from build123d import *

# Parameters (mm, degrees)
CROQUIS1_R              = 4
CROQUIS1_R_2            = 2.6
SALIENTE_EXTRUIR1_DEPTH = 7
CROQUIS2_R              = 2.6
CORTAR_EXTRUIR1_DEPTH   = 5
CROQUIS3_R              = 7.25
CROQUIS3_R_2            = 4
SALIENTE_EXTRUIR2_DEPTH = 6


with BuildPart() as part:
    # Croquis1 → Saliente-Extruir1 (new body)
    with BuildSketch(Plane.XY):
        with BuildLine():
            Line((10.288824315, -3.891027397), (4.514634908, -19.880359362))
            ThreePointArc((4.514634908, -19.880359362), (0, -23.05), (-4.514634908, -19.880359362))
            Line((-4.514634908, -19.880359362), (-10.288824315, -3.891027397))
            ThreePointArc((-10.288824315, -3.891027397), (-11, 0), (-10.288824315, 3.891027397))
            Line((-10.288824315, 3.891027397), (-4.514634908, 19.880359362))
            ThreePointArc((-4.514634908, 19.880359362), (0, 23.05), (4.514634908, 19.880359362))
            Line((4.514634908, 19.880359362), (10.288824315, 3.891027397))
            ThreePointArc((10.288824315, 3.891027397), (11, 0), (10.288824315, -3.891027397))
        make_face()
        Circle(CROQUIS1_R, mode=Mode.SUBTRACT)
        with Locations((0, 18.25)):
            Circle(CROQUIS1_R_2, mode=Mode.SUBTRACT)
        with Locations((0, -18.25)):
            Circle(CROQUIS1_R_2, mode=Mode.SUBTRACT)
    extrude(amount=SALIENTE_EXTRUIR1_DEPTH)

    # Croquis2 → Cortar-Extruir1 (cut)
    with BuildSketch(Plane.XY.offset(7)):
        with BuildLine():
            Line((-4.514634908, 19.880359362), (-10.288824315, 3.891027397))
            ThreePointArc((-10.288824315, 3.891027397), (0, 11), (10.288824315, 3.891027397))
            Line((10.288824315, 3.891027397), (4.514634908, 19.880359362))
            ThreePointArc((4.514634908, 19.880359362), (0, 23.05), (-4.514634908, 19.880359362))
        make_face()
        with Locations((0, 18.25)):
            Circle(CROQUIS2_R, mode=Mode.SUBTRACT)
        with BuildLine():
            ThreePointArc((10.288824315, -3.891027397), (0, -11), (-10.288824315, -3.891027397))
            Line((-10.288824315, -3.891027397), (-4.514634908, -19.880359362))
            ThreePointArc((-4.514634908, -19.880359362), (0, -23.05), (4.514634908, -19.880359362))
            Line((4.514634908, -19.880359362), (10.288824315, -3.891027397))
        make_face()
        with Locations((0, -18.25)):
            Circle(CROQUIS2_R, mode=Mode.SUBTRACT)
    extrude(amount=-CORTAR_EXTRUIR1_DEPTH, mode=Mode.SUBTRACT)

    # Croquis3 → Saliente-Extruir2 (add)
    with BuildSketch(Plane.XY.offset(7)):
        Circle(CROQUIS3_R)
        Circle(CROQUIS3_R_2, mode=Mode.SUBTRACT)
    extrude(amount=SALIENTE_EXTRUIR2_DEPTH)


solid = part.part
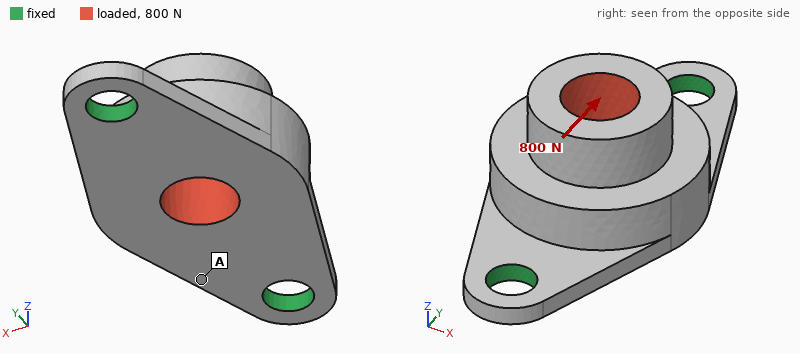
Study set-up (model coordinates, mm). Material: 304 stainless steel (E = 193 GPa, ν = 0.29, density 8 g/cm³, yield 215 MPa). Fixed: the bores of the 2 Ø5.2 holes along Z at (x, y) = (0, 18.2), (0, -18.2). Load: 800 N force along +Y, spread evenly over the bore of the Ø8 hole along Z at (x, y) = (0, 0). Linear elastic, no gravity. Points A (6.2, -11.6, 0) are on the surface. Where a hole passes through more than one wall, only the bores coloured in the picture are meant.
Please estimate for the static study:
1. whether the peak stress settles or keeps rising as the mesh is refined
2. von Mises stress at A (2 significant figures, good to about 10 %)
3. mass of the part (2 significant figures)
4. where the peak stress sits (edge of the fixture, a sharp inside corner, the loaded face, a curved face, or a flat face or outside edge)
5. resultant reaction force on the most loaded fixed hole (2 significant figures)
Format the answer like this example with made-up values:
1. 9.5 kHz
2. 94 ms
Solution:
1. keeps rising
2. 16 MPa
3. 28 g
4. edge of the fixture
5. 430 N
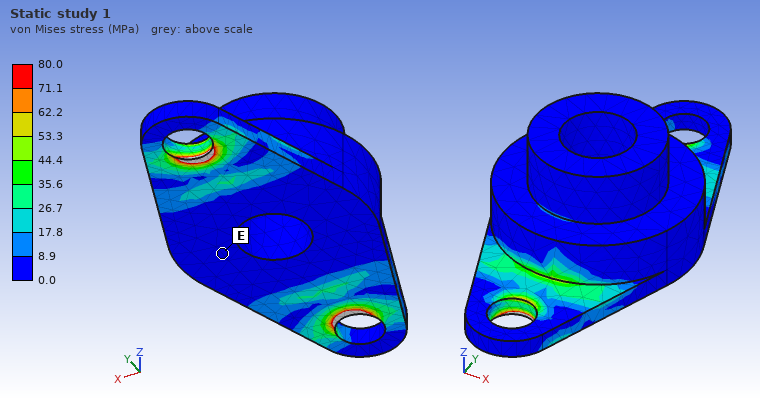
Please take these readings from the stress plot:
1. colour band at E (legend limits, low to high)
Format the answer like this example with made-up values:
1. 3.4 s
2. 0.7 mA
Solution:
1. 0.0 to 8.9 MPa
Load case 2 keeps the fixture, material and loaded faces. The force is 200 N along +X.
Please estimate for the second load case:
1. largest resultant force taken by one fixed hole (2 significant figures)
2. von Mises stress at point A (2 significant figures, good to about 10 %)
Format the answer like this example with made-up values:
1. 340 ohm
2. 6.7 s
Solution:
1. 100 N
2. 23 MPa
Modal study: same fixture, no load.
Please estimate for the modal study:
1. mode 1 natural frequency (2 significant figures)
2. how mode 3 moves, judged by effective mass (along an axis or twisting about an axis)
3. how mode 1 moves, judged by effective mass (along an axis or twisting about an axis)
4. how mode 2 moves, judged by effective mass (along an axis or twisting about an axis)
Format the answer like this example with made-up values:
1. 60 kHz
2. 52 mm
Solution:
1. 4500 Hz
2. along Y
3. along X
4. along Z
